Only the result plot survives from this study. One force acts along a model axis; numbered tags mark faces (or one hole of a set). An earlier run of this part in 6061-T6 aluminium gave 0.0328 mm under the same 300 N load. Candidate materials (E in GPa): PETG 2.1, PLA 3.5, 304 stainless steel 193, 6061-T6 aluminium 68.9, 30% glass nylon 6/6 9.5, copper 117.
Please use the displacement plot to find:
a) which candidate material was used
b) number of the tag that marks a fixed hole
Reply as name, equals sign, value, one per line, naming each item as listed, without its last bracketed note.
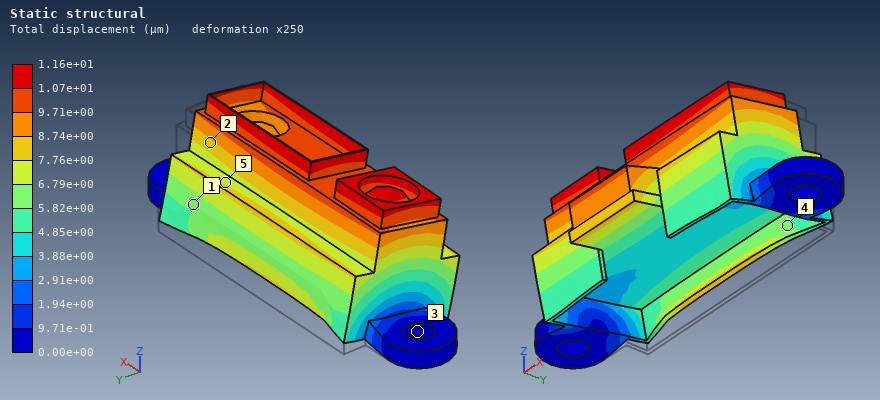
which candidate material was used = 304 stainless steel
number of the tag that marks a fixed hole = 3
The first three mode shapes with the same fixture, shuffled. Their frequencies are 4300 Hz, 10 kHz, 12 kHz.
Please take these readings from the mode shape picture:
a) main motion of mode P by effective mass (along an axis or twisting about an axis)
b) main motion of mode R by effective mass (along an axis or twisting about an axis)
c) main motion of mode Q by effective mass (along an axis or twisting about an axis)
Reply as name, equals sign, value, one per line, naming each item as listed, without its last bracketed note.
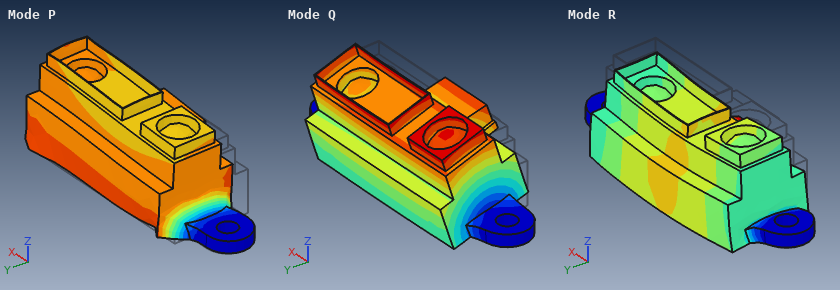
main motion of mode P by effective mass = along X
main motion of mode R by effective mass = along Z
main motion of mode Q by effective mass = along Y
